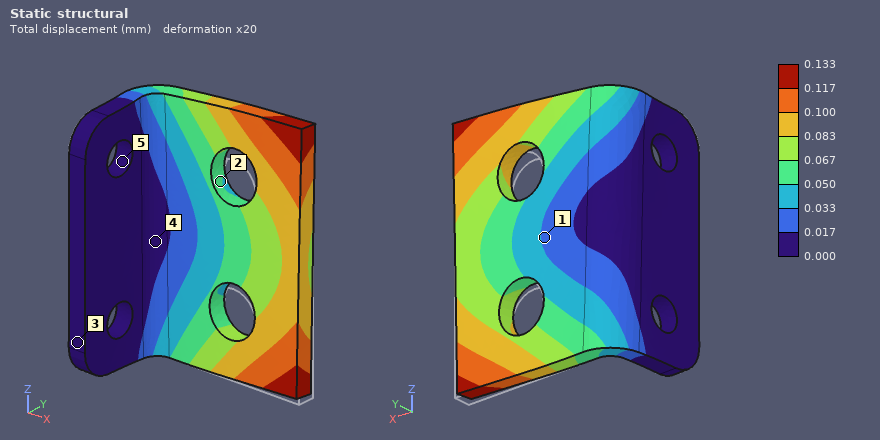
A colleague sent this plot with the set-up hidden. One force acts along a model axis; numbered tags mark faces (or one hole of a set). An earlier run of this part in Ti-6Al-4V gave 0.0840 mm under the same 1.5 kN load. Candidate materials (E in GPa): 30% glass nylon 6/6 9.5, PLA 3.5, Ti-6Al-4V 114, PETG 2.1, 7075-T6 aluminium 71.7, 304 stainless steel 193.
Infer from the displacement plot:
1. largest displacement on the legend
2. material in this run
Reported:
0.133 mm
7075-T6 aluminium
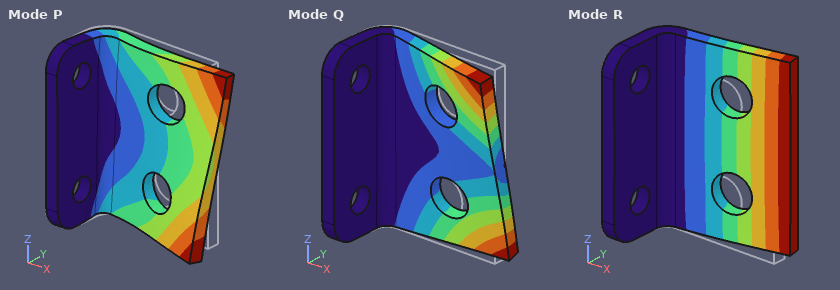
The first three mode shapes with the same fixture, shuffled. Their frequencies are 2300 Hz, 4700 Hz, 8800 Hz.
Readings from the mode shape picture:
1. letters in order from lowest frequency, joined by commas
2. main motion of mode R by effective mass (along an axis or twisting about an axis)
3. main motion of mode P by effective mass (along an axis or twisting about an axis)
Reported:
R, Q, P
along Y
along Z
